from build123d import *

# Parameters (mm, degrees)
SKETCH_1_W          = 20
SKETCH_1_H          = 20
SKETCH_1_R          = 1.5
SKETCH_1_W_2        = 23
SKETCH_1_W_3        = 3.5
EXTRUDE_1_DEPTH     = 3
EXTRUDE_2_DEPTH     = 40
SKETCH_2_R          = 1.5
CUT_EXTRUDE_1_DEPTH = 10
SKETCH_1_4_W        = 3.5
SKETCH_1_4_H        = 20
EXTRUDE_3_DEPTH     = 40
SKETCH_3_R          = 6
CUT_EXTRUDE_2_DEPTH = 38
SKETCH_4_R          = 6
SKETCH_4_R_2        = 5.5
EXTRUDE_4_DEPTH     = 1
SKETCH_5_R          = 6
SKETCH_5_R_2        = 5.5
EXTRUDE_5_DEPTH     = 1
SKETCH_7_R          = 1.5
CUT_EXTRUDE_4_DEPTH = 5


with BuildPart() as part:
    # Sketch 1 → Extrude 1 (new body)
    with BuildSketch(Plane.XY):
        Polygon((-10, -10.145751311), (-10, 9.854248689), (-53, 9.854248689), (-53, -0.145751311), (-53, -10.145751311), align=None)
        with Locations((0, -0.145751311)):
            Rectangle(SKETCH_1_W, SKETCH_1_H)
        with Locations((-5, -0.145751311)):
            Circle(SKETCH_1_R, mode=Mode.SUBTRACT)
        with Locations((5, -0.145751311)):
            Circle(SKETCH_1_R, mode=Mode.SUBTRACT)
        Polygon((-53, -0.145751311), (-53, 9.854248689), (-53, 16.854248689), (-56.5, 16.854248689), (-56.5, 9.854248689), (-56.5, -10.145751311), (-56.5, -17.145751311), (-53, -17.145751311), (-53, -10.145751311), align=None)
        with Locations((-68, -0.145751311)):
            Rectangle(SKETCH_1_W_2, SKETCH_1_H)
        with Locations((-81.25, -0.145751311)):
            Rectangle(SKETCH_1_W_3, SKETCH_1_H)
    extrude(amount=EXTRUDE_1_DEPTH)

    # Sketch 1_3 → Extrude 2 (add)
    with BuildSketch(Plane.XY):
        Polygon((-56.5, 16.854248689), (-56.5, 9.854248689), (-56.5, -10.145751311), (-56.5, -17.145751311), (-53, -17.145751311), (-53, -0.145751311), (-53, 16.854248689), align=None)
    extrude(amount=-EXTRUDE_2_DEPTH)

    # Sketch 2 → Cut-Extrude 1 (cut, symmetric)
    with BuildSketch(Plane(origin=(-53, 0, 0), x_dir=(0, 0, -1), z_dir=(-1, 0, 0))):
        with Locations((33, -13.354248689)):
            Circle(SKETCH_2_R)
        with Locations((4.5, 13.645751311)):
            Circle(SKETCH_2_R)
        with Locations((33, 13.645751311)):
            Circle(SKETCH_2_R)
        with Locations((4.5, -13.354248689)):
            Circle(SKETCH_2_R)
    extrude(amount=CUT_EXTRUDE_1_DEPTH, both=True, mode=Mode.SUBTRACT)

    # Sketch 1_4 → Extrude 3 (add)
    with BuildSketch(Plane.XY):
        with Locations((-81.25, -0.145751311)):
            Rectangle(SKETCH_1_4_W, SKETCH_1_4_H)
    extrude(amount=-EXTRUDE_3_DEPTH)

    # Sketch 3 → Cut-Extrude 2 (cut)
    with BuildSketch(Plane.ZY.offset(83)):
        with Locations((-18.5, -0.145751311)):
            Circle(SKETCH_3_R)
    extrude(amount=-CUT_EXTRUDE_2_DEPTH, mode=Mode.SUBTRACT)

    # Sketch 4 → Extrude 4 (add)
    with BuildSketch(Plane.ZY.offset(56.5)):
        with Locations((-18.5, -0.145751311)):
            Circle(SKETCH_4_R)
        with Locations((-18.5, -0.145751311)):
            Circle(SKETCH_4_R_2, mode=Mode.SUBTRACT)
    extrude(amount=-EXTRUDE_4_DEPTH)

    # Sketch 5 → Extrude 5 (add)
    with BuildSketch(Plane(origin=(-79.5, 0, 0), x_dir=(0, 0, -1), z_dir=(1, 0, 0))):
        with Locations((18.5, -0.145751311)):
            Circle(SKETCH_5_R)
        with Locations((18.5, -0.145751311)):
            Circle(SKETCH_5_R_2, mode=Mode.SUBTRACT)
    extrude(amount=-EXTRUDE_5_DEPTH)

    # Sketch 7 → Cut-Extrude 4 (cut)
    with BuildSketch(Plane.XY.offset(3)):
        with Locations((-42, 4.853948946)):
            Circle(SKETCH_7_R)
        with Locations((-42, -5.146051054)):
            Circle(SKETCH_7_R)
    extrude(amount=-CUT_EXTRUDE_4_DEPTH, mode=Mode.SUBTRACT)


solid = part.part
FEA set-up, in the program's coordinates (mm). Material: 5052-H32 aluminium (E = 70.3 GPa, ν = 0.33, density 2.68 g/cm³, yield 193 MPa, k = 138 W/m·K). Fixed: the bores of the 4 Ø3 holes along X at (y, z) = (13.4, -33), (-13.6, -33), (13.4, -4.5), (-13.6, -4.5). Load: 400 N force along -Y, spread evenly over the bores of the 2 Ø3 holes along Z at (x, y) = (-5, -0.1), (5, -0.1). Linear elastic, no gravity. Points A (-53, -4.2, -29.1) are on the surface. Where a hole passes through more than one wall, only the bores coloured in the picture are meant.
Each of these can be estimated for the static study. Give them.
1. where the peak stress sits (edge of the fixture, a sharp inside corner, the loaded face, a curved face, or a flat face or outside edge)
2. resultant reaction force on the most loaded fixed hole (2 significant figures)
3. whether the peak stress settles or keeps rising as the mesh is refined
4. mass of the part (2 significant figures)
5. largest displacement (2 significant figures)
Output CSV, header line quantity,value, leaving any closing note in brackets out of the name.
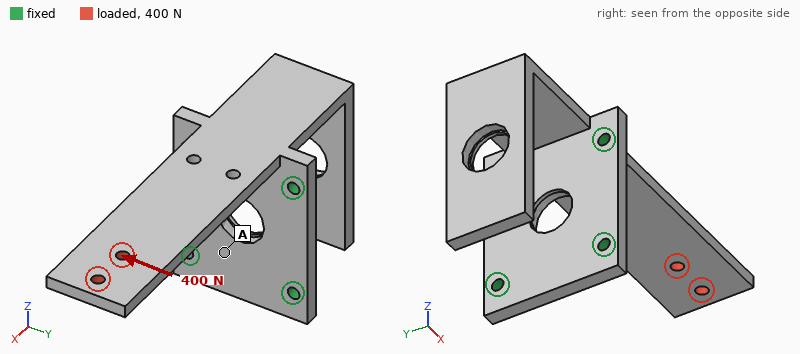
quantity,value
where the peak stress sits,edge of the fixture
resultant reaction force on the most loaded fixed hole,990 N
whether the peak stress settles or keeps rising as the mesh is refined,keeps rising
mass of the part,33 g
largest displacement,0.41 mm
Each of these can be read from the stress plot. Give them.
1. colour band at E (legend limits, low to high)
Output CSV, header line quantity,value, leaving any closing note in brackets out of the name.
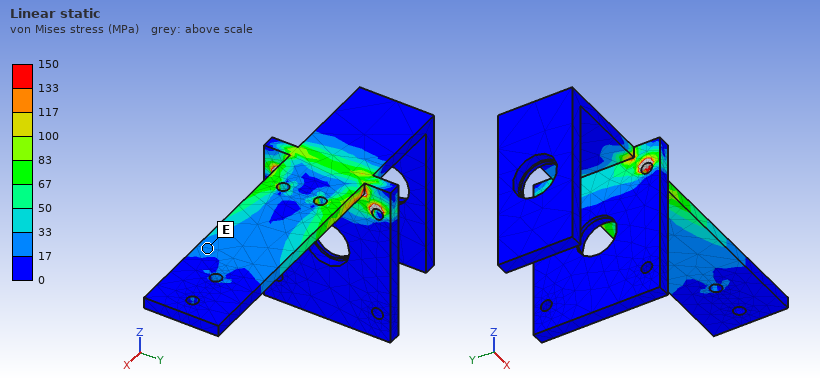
quantity,value
colour band at E,17 to 33 MPa
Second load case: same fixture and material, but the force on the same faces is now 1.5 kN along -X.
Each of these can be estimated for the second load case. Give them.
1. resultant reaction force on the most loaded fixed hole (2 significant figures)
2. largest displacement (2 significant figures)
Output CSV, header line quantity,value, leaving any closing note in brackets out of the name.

quantity,value
resultant reaction force on the most loaded fixed hole,790 N
largest displacement,0.31 mm
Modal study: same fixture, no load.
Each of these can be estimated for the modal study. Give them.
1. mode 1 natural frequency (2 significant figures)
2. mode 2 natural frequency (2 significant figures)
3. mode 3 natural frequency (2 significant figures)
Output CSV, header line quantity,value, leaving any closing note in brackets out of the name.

quantity,value
mode 1 natural frequency,550 Hz
mode 2 natural frequency,700 Hz
mode 3 natural frequency,1100 Hz
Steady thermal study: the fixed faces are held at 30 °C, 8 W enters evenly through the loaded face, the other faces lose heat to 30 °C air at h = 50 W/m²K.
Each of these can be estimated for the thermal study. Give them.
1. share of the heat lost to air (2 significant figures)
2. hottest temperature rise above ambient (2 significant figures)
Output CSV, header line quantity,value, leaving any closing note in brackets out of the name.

quantity,value
share of the heat lost to air,48 %
hottest temperature rise above ambient,41 K
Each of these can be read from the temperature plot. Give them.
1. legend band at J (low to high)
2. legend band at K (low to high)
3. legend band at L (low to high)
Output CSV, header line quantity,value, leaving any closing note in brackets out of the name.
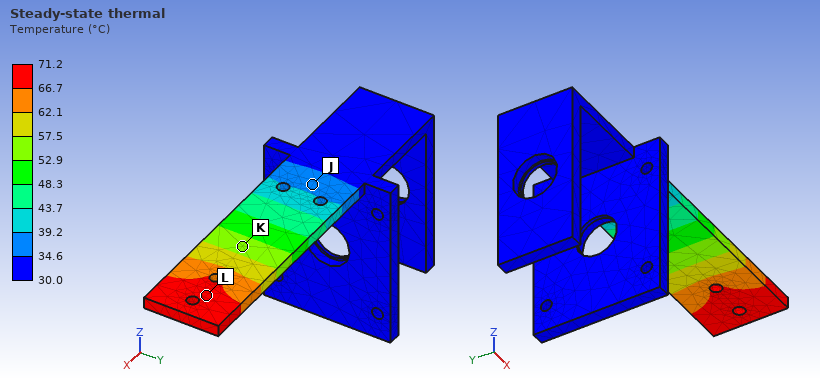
quantity,value
legend band at J,34.6 to 39.2 °C
legend band at K,52.9 to 57.5 °C
legend band at L,66.7 to 71.2 °C
